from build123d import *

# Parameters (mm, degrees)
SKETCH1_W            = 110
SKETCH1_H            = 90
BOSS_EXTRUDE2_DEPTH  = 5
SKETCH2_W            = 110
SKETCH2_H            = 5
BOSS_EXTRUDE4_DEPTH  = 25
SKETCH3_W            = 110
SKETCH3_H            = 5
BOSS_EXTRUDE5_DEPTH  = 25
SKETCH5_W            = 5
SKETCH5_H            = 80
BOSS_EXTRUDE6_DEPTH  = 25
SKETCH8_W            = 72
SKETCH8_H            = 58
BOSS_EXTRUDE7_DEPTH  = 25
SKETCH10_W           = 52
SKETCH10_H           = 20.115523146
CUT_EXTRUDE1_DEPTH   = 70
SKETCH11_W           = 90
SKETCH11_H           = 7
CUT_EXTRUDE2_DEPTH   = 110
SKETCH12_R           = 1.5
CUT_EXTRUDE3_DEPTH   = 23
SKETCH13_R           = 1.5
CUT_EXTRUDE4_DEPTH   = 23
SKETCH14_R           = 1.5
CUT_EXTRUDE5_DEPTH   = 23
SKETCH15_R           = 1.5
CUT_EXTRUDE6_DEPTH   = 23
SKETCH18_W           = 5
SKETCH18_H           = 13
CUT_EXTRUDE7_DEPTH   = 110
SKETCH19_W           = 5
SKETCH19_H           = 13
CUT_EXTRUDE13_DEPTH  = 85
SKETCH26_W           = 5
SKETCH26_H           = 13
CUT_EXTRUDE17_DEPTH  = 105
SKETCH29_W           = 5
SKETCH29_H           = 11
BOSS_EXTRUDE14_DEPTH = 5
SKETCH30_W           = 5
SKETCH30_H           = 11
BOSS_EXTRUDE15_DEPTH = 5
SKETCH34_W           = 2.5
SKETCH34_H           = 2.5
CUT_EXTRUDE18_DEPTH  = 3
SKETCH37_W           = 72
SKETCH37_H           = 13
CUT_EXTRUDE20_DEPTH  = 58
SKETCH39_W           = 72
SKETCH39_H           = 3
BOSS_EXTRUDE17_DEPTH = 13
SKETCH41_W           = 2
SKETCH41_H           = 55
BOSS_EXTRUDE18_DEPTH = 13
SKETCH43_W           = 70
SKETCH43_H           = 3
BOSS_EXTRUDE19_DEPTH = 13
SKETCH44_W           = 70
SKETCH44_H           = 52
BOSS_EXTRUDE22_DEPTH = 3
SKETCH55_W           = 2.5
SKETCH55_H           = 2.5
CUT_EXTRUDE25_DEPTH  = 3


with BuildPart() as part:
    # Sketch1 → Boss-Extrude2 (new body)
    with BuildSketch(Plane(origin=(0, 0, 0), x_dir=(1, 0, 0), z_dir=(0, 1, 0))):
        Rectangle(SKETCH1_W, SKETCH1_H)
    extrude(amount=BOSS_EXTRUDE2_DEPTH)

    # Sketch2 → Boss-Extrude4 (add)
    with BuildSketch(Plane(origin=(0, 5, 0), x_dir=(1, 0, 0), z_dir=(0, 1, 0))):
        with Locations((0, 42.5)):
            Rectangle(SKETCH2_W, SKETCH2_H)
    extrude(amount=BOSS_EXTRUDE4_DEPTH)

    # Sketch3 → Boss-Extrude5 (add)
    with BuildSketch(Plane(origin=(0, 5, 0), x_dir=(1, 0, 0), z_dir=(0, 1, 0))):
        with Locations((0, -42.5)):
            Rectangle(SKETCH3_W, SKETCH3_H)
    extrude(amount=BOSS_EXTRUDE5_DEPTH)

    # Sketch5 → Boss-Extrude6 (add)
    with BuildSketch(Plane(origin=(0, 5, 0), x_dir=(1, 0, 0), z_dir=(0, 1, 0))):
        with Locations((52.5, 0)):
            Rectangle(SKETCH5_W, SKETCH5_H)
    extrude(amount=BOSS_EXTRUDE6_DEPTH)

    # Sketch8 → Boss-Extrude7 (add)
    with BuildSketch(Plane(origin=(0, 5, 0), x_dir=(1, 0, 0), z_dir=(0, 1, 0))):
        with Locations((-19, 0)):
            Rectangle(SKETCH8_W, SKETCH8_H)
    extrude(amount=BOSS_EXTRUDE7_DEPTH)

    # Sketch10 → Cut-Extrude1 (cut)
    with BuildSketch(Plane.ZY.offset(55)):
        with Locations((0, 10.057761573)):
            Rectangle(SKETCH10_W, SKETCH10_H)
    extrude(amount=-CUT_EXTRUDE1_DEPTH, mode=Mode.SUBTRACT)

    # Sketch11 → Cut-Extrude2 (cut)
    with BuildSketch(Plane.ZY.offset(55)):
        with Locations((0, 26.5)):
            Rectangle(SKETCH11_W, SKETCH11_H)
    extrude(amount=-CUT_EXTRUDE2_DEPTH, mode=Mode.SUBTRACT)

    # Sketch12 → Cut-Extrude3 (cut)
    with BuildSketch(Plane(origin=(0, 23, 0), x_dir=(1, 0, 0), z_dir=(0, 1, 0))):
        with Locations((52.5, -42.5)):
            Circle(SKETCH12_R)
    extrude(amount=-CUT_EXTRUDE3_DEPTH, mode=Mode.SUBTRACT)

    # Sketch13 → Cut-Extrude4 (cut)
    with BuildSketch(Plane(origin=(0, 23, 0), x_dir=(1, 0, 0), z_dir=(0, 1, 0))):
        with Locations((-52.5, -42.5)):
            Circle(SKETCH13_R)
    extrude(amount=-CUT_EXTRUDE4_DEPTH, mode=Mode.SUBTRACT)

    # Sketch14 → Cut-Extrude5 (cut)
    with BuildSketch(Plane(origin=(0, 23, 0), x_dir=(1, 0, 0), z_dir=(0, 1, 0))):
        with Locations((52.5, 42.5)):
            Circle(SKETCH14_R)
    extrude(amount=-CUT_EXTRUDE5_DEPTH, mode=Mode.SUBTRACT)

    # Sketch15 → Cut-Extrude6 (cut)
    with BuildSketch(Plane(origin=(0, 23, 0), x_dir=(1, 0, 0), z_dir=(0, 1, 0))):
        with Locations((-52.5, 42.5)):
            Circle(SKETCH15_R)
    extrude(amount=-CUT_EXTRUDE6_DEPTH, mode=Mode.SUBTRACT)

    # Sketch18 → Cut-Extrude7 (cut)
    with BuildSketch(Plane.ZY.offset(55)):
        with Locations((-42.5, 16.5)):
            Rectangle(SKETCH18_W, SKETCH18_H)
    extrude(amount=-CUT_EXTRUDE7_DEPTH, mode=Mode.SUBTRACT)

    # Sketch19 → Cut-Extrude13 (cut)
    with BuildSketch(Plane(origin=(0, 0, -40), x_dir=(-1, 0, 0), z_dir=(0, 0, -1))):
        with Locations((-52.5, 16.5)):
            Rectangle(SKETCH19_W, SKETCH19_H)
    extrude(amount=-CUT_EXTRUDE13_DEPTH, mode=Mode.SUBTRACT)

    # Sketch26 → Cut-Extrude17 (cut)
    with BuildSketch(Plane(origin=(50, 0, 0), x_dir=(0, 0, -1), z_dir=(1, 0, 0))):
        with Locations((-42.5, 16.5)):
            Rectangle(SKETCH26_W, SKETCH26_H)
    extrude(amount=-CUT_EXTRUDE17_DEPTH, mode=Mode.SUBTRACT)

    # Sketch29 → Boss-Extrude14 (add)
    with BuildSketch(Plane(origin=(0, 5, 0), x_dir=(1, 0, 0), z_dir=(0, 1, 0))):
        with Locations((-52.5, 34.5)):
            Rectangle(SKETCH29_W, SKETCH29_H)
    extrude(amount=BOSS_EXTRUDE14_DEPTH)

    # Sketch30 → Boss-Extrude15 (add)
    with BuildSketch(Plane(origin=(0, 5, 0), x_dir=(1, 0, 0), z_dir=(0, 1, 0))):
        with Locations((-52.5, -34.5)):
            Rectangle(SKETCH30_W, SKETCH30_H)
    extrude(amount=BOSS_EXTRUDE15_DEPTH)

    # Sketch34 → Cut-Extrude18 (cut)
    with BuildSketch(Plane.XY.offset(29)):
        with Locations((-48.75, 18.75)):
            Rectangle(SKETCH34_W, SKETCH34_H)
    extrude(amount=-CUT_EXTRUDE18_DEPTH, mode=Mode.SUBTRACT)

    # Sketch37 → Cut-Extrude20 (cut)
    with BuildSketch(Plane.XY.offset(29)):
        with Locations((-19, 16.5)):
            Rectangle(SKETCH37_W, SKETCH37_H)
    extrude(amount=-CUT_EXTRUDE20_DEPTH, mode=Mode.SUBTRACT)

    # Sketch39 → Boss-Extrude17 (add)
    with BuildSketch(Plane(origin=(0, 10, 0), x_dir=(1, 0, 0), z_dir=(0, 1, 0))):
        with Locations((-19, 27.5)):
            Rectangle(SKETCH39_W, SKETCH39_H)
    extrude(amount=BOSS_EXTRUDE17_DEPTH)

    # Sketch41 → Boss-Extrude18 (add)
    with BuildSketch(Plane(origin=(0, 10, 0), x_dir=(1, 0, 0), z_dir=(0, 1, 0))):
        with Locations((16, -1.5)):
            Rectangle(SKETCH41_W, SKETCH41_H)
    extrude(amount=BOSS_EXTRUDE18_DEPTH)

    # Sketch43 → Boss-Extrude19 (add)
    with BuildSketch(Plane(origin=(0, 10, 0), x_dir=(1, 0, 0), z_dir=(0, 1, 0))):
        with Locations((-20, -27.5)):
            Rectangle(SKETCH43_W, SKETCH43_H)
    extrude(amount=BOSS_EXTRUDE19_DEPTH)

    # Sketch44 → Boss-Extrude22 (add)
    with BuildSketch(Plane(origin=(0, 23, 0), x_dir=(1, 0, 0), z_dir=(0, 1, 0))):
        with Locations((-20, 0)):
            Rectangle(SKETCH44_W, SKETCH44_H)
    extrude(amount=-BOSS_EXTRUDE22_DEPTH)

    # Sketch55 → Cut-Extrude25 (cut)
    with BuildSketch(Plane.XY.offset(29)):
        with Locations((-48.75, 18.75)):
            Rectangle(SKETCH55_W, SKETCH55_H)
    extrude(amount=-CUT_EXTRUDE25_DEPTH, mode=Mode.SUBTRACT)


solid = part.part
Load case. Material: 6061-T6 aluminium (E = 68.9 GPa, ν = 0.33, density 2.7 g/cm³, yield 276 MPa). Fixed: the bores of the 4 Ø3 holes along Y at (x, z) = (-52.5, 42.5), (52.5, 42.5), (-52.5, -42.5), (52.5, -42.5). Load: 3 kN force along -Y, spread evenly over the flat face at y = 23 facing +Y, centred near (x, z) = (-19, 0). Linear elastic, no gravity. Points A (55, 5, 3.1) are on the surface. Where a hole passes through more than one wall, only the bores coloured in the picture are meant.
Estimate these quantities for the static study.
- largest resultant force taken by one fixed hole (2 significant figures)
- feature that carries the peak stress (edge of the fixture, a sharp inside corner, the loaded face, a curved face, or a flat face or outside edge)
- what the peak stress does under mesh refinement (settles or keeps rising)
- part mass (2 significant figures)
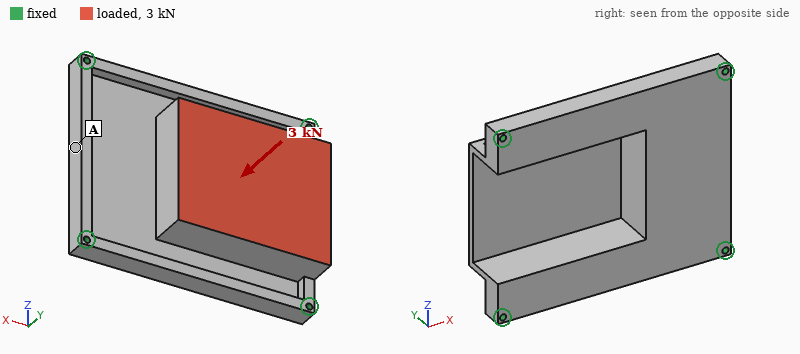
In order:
1.2 kN
edge of the fixture
keeps rising
160 g
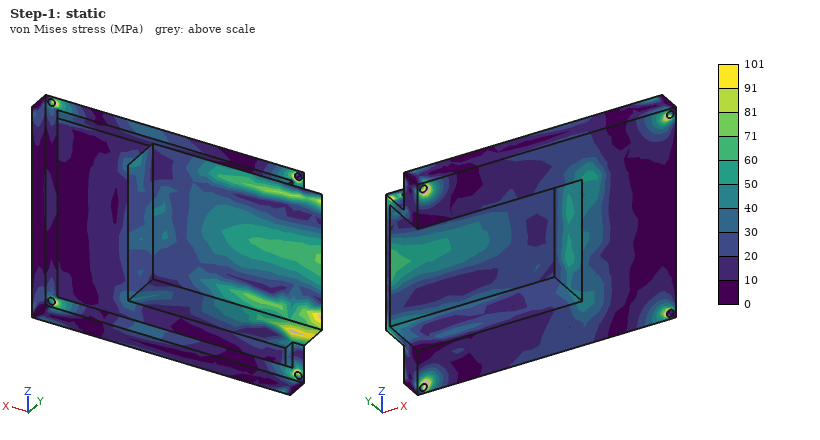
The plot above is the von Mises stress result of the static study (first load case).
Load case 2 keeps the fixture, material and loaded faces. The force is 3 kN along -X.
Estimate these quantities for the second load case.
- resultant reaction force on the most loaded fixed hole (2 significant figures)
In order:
1000 N
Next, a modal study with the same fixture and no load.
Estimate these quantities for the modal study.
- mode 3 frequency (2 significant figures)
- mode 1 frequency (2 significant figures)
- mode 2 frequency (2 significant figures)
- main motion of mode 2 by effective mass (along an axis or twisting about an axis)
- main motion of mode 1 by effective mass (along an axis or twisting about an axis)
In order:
4700 Hz
2700 Hz
3700 Hz
along Z
along Y
